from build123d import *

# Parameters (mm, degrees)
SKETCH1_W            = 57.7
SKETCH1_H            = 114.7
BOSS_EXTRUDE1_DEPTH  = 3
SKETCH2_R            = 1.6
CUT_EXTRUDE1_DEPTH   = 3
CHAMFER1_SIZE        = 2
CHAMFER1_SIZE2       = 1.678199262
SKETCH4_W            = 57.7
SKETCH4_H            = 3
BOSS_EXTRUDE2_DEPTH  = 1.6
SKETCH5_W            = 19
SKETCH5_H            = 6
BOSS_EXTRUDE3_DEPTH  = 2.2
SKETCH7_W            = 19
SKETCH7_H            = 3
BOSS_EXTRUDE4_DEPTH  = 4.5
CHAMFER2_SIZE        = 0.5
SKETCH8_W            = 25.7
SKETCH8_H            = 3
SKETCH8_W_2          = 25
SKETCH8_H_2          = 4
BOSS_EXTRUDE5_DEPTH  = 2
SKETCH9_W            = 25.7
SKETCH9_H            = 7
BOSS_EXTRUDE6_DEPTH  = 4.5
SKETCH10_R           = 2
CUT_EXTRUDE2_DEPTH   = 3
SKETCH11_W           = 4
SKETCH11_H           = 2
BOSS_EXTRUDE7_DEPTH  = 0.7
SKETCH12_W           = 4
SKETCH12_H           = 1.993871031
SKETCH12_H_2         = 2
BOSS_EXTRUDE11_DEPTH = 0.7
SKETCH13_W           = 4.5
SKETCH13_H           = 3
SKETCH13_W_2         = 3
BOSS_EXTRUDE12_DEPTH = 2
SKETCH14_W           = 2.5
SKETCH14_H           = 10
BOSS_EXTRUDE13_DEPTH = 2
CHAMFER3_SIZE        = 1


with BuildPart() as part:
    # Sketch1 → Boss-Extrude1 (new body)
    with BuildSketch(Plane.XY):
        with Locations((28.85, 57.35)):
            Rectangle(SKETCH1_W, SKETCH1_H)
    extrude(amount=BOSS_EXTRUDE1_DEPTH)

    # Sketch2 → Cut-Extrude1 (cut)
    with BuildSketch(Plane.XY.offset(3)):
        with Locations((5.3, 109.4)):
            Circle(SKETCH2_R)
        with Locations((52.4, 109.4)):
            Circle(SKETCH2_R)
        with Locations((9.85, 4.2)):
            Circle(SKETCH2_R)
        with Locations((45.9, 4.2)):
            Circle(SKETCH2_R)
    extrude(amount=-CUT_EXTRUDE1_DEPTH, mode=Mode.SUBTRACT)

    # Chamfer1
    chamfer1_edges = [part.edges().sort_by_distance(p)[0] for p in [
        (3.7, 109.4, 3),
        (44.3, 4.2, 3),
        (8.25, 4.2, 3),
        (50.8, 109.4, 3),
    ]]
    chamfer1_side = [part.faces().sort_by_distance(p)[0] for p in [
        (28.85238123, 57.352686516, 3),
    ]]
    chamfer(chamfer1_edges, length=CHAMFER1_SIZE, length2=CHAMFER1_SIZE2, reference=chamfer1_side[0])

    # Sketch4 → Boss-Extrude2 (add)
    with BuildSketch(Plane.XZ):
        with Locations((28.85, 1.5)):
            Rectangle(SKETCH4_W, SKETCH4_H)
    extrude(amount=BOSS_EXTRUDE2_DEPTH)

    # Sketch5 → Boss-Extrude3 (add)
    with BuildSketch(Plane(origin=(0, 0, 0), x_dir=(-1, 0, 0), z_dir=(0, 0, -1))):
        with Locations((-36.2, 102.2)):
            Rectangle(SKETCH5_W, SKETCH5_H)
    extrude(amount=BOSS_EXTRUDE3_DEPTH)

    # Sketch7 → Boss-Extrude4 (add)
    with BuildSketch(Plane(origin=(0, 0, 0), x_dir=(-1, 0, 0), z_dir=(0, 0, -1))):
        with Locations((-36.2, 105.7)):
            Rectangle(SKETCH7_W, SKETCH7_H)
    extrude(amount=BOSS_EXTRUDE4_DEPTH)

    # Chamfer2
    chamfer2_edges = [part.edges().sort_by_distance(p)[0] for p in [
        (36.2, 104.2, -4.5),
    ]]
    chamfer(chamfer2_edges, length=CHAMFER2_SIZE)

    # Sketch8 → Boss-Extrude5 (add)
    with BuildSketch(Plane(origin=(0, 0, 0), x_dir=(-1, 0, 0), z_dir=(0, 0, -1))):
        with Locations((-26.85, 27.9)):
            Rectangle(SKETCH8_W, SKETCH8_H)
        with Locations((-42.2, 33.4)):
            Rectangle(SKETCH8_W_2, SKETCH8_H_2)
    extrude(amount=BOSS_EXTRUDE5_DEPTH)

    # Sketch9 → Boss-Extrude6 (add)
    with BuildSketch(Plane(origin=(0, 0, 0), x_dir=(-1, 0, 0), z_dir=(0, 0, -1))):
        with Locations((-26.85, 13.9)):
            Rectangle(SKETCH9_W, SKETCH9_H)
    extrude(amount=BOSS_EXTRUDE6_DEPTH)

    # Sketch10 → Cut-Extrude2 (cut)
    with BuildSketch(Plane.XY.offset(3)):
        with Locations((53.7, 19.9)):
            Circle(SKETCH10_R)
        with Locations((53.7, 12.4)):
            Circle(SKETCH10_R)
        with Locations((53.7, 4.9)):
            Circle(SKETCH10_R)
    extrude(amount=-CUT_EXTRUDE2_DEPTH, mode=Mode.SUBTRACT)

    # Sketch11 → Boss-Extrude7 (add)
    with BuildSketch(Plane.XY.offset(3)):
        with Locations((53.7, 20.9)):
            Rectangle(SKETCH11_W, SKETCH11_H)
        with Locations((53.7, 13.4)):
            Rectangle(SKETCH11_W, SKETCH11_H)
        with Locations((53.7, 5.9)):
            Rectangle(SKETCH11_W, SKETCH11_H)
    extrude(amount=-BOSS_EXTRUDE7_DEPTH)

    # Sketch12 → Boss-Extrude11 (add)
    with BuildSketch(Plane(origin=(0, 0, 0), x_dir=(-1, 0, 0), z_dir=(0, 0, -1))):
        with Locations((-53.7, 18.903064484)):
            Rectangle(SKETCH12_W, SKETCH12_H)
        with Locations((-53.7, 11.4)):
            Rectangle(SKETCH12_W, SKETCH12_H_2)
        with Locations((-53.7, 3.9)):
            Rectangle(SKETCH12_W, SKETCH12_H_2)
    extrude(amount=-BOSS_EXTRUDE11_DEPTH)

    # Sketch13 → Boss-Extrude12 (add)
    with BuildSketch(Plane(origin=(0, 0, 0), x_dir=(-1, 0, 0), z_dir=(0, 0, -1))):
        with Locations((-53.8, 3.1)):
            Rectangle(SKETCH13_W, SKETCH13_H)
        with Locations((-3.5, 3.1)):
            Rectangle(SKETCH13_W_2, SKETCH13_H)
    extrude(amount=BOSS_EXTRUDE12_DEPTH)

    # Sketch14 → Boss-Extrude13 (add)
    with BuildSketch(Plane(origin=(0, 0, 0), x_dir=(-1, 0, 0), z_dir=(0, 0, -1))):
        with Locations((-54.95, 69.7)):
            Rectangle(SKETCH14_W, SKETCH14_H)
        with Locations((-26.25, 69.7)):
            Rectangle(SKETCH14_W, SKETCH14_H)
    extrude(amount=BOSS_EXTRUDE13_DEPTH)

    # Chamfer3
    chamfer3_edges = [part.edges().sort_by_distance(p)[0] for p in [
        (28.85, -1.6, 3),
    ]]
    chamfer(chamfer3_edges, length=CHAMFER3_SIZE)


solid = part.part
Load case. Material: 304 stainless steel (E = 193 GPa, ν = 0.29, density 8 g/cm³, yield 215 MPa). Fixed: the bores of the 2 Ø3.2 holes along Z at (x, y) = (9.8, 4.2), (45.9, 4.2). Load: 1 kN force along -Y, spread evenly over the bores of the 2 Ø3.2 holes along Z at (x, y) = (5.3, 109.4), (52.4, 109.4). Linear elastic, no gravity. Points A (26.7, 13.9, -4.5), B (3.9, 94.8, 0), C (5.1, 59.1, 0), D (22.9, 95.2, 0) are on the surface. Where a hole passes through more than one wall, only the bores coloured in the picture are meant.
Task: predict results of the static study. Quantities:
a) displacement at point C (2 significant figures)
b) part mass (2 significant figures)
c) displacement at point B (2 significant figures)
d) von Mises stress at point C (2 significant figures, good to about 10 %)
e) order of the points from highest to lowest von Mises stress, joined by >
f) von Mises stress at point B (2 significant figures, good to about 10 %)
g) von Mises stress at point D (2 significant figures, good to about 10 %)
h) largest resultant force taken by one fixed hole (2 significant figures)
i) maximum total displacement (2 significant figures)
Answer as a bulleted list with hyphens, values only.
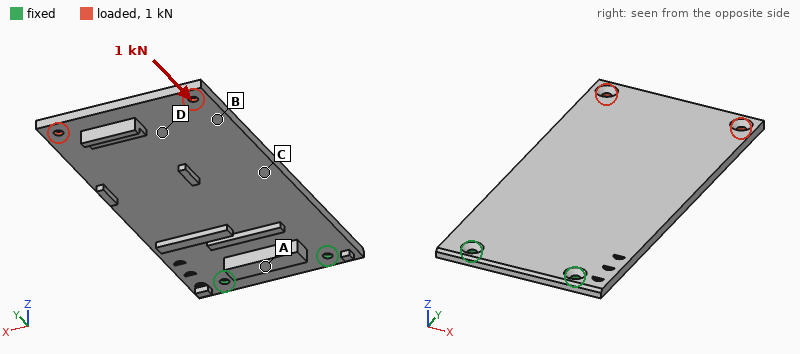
- 0.045 mm
- 170 g
- 0.12 mm
- 15 MPa
- B > C > D > A
- 21 MPa
- 11 MPa
- 530 N
- 0.19 mm
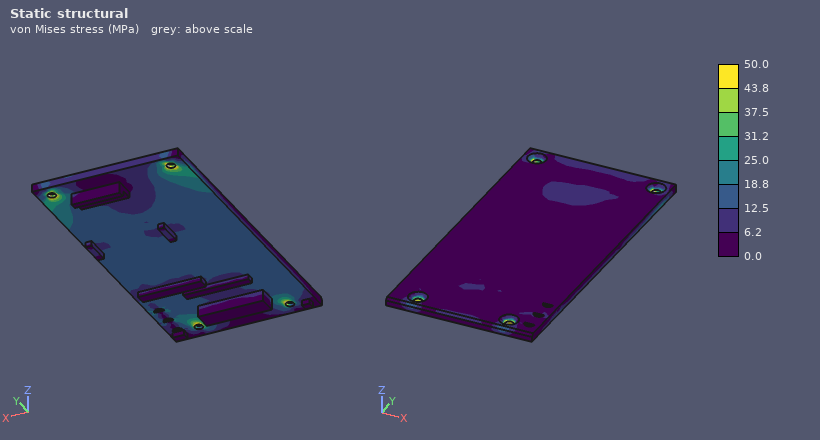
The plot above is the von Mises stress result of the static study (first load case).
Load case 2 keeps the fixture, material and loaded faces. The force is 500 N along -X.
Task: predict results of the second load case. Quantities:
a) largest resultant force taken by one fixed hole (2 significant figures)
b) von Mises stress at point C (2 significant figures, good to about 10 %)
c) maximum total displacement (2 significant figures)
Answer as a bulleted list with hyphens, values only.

- 1.4 kN
- 14 MPa
- 56 µm
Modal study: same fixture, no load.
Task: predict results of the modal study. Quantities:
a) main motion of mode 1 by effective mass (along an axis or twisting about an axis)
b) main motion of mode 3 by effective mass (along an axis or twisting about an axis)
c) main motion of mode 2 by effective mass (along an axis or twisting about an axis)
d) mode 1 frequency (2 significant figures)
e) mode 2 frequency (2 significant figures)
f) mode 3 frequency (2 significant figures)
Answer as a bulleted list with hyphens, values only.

- along Z
- along Z
- twisting about Y
- 170 Hz
- 830 Hz
- 1100 Hz
